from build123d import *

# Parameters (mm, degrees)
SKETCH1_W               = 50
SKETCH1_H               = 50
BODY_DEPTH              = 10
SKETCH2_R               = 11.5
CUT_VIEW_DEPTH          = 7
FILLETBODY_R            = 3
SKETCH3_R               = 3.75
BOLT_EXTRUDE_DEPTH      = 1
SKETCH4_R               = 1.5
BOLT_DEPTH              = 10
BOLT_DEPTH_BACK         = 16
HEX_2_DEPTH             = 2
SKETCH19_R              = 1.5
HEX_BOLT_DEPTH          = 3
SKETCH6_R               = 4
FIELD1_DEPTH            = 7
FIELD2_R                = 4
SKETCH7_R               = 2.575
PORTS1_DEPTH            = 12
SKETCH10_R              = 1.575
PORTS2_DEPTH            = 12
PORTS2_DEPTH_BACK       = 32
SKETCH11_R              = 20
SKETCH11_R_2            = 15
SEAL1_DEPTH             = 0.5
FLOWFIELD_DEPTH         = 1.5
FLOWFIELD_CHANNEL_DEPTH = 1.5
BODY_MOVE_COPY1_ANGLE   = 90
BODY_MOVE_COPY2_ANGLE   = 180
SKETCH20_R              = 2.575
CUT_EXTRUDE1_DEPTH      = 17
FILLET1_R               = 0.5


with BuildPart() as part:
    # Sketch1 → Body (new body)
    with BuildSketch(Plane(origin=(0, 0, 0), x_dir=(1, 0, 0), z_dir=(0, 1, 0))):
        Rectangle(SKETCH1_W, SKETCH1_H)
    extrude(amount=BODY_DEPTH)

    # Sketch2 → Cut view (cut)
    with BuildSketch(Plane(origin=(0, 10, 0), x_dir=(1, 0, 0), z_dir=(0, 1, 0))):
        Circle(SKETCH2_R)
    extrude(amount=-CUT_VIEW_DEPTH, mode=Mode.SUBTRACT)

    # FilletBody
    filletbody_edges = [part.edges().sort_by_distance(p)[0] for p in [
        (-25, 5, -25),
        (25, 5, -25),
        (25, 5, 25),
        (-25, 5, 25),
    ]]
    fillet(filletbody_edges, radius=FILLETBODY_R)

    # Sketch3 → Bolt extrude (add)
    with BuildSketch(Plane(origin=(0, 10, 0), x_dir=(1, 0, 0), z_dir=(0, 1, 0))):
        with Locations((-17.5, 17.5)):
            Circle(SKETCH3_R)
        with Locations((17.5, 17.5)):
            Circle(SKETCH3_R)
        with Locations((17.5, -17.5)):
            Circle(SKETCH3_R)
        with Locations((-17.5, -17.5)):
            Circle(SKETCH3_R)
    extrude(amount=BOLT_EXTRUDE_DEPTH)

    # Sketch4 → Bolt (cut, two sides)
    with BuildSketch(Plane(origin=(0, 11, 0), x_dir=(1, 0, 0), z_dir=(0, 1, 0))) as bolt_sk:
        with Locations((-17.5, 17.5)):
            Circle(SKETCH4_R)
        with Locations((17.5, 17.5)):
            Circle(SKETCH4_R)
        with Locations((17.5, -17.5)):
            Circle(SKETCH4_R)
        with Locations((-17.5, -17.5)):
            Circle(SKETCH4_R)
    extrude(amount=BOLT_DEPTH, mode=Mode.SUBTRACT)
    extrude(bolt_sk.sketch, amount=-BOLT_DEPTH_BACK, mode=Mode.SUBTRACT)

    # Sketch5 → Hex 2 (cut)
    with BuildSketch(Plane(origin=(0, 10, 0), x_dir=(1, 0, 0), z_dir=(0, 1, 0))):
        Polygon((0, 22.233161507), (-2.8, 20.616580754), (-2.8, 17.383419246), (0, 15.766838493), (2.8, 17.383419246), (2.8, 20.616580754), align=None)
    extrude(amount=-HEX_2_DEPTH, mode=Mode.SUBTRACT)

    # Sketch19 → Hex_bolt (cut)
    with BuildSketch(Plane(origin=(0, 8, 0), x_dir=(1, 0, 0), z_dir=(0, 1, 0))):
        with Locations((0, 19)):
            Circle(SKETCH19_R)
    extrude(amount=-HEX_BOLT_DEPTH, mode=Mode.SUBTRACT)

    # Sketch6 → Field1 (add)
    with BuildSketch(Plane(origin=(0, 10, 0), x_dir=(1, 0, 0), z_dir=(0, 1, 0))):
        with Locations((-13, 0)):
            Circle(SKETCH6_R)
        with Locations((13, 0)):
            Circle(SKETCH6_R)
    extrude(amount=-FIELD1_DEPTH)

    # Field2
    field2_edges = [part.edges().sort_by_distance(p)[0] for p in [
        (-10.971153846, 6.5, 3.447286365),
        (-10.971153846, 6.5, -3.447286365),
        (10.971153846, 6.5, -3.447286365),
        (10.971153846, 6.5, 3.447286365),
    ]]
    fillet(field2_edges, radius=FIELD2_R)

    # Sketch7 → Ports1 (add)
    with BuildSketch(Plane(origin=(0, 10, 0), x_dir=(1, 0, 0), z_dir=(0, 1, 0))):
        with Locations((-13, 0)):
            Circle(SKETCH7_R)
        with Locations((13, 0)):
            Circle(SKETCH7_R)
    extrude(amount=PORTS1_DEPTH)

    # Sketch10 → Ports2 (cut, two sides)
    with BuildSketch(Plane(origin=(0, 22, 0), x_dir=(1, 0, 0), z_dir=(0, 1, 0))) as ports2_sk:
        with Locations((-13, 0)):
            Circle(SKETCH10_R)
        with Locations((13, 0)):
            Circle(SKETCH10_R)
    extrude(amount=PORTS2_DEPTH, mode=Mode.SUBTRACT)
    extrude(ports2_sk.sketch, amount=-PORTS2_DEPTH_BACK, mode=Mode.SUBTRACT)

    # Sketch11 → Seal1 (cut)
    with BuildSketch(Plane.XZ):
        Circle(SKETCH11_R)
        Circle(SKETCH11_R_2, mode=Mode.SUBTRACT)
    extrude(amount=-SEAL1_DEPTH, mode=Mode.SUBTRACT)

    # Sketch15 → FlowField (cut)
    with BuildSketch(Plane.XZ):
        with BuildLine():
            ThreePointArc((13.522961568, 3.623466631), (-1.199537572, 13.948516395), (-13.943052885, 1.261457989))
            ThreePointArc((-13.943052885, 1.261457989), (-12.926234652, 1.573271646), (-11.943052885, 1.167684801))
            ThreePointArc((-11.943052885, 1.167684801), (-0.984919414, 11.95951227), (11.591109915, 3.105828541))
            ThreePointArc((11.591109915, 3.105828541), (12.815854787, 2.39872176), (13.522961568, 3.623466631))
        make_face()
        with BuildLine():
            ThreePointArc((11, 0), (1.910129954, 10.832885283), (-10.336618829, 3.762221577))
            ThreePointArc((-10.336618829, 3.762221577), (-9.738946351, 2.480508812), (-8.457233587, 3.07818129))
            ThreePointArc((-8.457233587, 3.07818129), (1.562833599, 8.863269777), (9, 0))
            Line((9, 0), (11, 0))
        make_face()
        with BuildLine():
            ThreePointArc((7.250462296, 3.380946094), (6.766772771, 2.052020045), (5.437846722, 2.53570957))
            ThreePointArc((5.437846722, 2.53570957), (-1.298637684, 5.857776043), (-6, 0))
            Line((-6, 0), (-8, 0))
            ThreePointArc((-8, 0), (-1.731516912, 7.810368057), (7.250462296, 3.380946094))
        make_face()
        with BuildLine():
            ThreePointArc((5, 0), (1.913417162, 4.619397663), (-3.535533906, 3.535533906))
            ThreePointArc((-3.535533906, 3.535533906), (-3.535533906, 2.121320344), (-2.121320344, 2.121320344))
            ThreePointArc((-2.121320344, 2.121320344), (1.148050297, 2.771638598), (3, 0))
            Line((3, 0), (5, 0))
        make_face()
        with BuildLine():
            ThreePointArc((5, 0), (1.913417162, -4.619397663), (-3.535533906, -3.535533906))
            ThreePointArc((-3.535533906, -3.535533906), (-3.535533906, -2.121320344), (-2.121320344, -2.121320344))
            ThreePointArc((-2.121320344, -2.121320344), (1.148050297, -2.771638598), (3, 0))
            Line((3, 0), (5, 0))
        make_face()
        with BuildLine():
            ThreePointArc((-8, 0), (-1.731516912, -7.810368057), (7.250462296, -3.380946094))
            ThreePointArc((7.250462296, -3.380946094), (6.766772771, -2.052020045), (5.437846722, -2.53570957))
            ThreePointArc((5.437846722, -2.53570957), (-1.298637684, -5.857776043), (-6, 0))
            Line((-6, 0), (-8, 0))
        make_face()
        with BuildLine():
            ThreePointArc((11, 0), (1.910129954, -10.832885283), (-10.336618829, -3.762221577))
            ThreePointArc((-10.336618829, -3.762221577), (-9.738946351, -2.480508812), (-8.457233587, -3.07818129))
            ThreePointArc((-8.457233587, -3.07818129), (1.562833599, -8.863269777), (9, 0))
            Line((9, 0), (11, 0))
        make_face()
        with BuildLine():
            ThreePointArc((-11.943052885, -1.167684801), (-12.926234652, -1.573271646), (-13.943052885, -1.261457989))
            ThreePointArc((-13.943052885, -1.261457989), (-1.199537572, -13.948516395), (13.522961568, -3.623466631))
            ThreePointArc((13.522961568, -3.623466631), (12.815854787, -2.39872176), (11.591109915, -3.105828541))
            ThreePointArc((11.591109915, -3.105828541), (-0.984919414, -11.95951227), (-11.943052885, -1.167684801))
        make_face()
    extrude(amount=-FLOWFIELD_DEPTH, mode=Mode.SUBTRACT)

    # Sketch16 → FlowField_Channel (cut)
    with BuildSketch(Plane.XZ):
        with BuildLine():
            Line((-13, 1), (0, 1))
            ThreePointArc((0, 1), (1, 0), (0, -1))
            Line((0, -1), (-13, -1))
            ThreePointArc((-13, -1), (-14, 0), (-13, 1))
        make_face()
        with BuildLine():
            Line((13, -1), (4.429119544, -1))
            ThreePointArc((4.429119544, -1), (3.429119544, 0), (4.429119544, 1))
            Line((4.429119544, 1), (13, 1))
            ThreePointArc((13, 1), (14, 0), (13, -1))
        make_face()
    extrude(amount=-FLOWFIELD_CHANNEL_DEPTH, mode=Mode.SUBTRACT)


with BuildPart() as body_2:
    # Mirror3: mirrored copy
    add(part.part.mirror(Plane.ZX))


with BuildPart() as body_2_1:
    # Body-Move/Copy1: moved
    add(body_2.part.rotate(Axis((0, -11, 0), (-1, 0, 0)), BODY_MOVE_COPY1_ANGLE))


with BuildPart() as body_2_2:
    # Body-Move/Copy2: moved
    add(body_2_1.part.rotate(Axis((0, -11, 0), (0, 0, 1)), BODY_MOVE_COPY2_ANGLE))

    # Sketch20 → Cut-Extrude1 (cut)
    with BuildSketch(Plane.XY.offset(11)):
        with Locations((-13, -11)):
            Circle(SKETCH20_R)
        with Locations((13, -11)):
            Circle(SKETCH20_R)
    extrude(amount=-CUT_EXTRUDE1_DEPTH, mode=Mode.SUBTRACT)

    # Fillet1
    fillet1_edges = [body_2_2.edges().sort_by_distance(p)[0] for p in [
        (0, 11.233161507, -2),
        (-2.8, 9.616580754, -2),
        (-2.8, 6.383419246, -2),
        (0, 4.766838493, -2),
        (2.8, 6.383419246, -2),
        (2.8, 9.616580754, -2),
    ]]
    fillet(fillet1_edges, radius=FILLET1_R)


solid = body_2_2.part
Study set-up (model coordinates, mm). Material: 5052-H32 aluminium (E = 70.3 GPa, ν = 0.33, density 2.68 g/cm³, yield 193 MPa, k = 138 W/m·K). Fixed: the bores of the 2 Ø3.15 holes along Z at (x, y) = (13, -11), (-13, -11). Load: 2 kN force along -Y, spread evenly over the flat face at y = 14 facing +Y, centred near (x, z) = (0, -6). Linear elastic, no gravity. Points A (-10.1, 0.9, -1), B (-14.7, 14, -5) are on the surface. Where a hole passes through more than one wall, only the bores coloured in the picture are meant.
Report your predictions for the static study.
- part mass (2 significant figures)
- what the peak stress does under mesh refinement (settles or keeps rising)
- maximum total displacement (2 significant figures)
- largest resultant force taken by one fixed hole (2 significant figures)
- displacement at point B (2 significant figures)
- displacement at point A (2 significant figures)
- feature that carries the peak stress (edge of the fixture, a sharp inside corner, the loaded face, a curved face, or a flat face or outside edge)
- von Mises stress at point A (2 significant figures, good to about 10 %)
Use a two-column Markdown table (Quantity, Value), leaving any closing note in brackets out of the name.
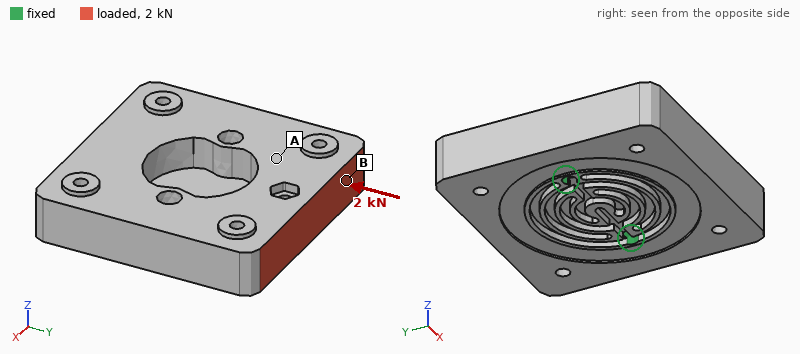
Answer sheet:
| Quantity | Value |
|---|---|
| part mass | 56 g |
| what the peak stress does under mesh refinement | keeps rising |
| maximum total displacement | 19 µm |
| largest resultant force taken by one fixed hole | 1.0 kN |
| displacement at point B | 17 µm |
| displacement at point A | 10 µm |
| feature that carries the peak stress | edge of the fixture |
| von Mises stress at point A | 8.6 MPa |
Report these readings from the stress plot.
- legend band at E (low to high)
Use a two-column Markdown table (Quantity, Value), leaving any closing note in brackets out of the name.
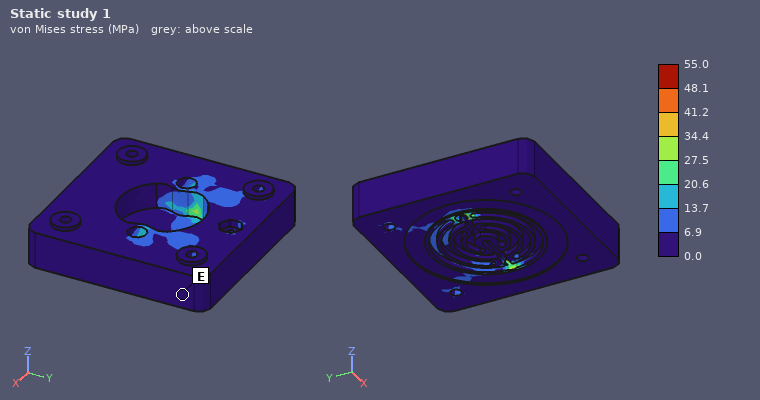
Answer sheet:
| Quantity | Value |
|---|---|
| legend band at E | 0.0 to 6.9 MPa |
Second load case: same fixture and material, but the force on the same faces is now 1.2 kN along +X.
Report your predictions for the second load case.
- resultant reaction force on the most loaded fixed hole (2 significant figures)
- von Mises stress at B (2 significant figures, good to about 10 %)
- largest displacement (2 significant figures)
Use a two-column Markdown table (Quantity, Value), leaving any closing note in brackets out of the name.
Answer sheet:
| Quantity | Value |
|---|---|
| resultant reaction force on the most loaded fixed hole | 1.2 kN |
| von Mises stress at B | 6.6 MPa |
| largest displacement | 12 µm |
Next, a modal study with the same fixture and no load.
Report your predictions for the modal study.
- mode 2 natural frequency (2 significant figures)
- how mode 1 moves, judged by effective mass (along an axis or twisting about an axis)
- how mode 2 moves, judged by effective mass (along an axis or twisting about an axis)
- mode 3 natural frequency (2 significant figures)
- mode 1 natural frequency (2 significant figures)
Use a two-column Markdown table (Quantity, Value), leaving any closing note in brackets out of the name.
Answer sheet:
| Quantity | Value |
|---|---|
| mode 2 natural frequency | 8500 Hz |
| how mode 1 moves, judged by effective mass | twisting about X |
| how mode 2 moves, judged by effective mass | along Z |
| mode 3 natural frequency | 9600 Hz |
| mode 1 natural frequency | 3600 Hz |
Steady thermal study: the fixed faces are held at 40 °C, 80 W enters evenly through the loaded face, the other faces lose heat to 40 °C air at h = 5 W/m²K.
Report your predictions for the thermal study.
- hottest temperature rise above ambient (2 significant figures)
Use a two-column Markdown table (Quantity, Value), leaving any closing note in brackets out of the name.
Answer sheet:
| Quantity | Value |
|---|---|
| hottest temperature rise above ambient | 53 K |
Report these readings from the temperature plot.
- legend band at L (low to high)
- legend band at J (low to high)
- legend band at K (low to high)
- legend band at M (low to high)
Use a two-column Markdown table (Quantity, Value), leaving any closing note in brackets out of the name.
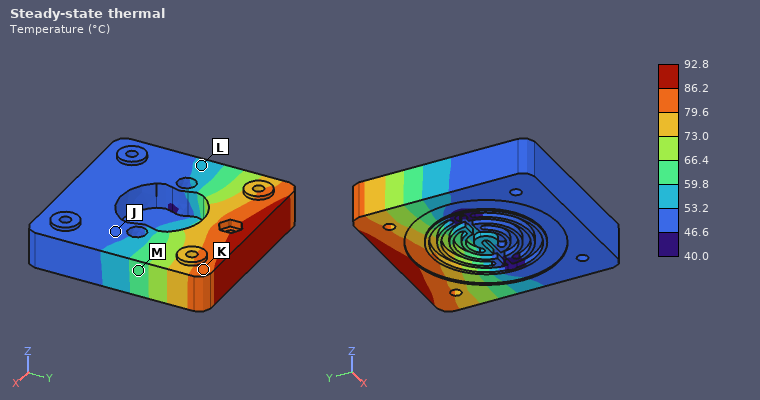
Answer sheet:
| Quantity | Value |
|---|---|
| legend band at L | 53.2 to 59.8 °C |
| legend band at J | 46.6 to 53.2 °C |
| legend band at K | 79.6 to 86.2 °C |
| legend band at M | 59.8 to 66.4 °C |
